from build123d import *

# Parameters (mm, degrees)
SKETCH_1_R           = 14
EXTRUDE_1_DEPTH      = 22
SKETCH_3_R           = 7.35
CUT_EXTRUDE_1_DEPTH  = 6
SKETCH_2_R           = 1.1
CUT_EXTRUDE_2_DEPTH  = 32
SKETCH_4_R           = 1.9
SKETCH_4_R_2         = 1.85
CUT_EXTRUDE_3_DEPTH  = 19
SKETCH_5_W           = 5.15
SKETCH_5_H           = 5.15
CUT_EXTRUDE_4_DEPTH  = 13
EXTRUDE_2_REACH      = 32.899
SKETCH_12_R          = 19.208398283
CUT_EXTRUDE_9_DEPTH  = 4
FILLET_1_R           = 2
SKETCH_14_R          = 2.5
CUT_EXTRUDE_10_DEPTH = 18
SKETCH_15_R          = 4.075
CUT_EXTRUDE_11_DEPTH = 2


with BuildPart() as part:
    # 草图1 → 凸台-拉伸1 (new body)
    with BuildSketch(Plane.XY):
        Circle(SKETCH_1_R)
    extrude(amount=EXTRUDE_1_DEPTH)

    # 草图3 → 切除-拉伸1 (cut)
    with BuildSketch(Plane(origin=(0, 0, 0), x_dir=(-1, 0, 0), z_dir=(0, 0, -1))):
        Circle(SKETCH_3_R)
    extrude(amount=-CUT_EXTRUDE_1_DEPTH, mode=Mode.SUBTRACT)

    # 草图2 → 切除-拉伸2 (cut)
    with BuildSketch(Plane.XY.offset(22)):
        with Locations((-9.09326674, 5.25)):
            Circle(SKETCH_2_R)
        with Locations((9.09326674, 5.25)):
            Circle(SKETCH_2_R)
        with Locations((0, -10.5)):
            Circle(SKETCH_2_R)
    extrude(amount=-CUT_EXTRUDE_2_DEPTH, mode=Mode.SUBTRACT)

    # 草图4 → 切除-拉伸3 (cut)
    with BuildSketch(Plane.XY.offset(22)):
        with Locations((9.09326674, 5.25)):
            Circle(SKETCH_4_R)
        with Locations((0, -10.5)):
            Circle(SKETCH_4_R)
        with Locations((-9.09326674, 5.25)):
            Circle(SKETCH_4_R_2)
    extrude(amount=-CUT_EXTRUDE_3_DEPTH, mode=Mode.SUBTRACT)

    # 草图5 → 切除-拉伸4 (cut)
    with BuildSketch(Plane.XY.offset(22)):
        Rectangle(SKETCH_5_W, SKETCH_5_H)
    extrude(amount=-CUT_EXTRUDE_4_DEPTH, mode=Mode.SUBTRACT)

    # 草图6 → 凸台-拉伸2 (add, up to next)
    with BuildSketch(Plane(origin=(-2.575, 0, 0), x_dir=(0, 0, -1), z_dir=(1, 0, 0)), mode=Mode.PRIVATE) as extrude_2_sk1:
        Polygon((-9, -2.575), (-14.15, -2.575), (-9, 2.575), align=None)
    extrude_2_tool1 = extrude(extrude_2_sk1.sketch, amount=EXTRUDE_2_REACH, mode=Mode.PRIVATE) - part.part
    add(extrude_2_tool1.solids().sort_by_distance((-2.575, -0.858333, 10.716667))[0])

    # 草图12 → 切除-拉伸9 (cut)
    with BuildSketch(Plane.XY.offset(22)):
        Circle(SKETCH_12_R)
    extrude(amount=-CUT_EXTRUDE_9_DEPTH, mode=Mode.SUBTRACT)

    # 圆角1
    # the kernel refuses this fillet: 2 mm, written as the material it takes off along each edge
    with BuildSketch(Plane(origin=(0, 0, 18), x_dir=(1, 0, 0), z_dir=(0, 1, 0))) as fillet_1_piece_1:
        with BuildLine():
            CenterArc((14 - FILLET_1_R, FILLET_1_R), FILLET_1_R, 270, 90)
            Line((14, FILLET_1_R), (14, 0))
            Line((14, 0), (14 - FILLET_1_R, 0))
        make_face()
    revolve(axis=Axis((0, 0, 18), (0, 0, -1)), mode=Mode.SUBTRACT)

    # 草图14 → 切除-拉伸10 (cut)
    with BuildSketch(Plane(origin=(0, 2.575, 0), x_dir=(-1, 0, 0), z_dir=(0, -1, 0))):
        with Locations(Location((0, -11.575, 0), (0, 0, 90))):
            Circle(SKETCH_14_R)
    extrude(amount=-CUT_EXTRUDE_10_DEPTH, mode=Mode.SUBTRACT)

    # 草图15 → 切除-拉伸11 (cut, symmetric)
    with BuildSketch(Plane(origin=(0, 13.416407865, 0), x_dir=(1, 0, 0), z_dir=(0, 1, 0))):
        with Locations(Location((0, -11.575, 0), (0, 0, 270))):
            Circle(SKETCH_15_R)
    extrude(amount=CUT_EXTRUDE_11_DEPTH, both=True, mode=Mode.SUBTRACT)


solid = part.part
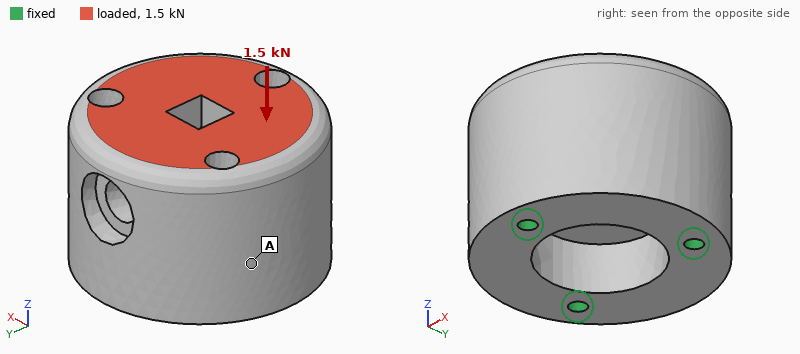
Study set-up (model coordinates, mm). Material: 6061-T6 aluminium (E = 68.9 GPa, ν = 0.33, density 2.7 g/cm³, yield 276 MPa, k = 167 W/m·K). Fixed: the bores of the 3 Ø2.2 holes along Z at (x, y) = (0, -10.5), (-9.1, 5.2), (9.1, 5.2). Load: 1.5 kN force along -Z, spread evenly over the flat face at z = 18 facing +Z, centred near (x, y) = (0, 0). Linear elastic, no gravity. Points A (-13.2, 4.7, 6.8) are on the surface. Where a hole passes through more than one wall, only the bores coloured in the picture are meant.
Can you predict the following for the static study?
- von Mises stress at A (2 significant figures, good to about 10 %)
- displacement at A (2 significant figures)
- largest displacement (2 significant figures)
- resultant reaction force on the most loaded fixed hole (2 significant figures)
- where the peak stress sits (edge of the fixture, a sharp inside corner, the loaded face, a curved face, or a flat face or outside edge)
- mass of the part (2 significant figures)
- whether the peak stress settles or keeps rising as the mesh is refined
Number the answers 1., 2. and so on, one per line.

1. 7.2 MPa
2. 1.7 µm
3. 3.0 µm
4. 510 N
5. edge of the fixture
6. 24 g
7. keeps rising
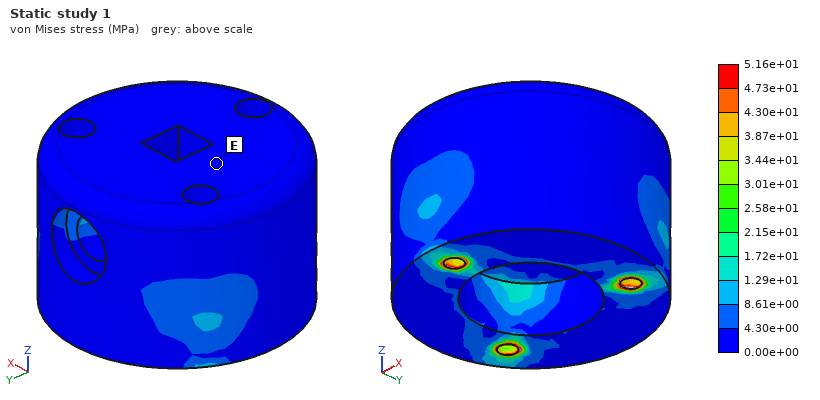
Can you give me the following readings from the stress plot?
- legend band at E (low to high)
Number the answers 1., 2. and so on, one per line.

1. 0.00e+00 to 4.30e+00 MPa
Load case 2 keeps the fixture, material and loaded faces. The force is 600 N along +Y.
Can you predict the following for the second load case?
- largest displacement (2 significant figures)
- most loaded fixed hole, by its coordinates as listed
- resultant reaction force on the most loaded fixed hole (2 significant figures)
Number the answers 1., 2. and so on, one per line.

1. 6.8 µm
2. (0, -10.5)
3. 610 N
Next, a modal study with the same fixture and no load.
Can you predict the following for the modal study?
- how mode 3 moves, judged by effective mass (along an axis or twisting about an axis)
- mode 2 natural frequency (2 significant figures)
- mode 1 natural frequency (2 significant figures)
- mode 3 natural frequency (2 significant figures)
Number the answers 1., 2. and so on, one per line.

1. along Z
2. 16 kHz
3. 15 kHz
4. 28 kHz
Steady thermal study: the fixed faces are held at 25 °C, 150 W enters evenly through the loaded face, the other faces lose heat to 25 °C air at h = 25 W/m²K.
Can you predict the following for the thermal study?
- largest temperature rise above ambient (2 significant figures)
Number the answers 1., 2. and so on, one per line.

1. 58 K
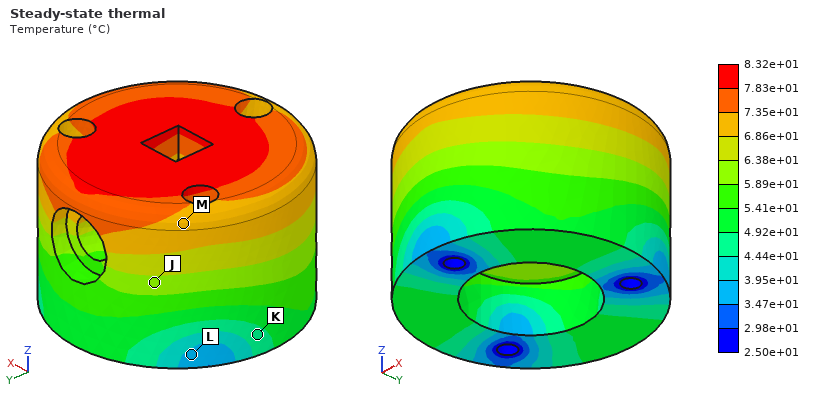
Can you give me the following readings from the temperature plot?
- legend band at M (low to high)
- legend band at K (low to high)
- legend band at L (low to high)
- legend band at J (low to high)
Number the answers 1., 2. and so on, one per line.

1. 6.86e+01 to 7.35e+01 °C
2. 4.44e+01 to 4.92e+01 °C
3. 3.47e+01 to 3.95e+01 °C
4. 5.89e+01 to 6.38e+01 °C
